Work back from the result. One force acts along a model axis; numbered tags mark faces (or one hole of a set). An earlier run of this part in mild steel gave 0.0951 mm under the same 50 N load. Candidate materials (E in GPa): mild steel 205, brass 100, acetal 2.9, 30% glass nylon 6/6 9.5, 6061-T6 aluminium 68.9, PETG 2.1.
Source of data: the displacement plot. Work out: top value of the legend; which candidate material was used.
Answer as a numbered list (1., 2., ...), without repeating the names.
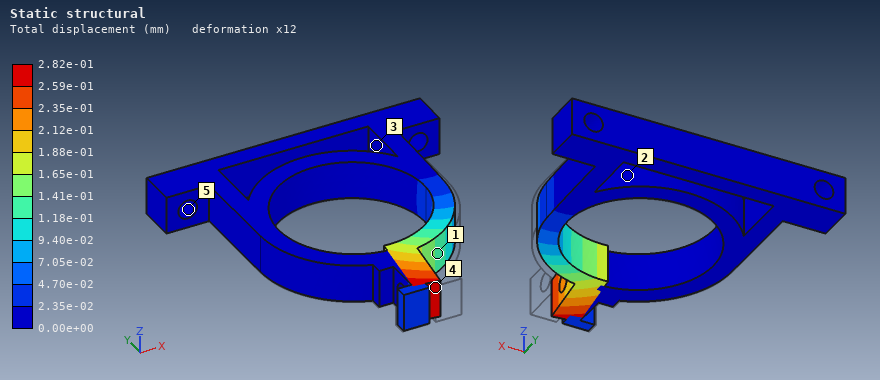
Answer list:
1. 2.82e-01 mm
2. 6061-T6 aluminium
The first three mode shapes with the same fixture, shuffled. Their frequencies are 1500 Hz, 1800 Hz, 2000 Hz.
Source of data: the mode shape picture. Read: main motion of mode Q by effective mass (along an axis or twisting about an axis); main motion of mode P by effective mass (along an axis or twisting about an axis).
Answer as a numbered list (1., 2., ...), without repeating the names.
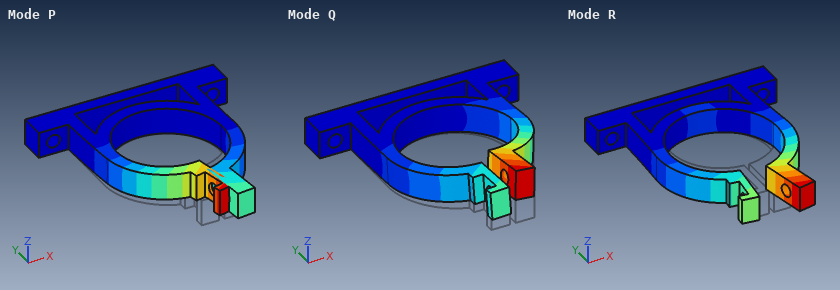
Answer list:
1. along Z
2. along X
